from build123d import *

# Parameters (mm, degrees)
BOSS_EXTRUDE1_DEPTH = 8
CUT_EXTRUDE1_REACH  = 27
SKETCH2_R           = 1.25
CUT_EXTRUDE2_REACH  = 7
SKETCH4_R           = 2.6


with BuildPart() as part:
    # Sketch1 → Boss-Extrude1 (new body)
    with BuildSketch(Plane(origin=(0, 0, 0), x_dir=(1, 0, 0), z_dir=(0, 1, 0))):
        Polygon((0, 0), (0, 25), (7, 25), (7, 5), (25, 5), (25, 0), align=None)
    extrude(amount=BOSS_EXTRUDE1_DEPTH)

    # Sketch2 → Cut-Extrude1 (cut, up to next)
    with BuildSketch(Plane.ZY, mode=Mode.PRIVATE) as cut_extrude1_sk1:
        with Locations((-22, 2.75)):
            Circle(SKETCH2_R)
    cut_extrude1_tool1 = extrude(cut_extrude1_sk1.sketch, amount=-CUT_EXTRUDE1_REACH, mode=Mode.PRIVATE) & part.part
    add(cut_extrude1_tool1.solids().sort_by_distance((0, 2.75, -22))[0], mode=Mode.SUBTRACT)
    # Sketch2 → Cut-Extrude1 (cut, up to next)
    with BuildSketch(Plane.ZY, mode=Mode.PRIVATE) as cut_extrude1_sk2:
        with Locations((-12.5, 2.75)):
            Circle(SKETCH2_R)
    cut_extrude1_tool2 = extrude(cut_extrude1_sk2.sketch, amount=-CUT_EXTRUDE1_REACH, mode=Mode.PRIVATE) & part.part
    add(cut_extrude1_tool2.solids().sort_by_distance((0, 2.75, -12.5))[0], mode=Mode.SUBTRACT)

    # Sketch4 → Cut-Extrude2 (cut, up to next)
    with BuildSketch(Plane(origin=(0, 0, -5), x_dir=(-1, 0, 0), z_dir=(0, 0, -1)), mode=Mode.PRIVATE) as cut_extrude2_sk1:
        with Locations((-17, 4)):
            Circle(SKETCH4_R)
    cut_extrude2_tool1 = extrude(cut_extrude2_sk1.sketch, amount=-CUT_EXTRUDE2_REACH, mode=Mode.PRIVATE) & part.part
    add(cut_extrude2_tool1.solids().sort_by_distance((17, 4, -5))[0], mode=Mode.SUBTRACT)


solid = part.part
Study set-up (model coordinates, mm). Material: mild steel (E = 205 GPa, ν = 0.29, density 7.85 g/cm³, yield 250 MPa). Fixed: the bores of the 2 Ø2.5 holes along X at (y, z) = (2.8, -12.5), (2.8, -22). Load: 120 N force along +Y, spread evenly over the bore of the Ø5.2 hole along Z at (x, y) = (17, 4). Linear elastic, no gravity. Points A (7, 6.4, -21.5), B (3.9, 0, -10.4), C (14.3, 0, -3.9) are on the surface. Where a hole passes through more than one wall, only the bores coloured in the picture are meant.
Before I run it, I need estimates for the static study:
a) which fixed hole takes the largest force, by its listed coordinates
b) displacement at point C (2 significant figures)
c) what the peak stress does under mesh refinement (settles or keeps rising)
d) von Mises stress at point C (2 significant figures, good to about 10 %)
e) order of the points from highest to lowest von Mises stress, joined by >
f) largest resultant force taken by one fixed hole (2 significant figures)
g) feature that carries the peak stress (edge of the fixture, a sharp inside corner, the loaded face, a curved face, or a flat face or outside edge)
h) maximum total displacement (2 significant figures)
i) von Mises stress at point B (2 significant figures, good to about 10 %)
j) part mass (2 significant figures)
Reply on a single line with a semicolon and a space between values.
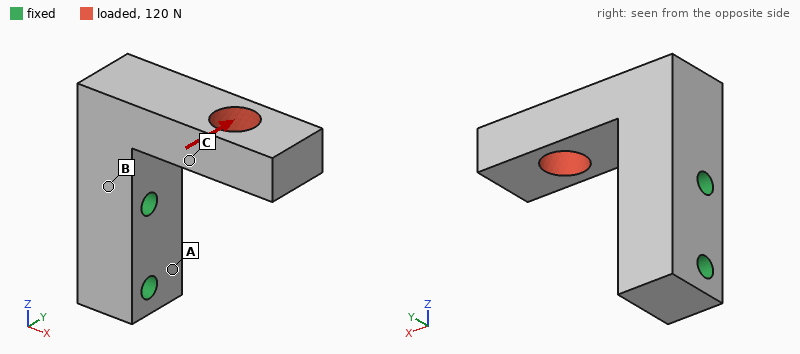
(2.8, -12.5); 7.3 µm; keeps rising; 18 MPa; B > C > A; 190 N; edge of the fixture; 15 µm; 33 MPa; 15 g
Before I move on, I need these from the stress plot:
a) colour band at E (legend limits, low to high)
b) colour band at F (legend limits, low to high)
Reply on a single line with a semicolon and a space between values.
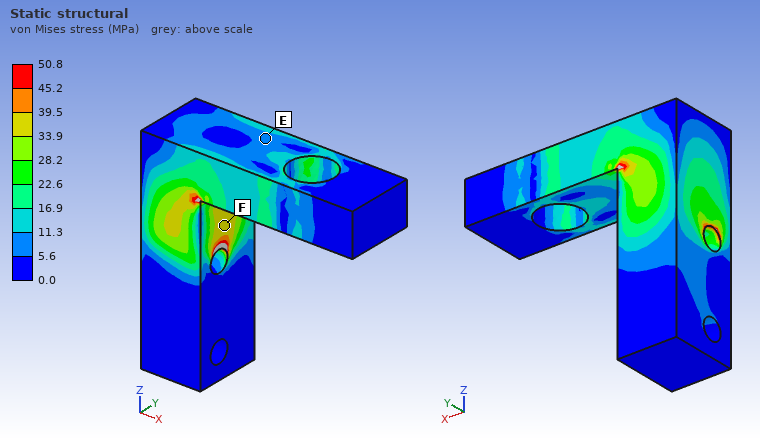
5.6 to 11.3 MPa; 33.9 to 39.5 MPa
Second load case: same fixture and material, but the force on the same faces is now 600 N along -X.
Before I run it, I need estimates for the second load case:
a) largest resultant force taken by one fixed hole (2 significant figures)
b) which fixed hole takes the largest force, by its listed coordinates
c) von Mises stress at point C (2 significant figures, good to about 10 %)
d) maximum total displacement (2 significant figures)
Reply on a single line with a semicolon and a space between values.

690 N; (2.8, -12.5); 23 MPa; 18 µm
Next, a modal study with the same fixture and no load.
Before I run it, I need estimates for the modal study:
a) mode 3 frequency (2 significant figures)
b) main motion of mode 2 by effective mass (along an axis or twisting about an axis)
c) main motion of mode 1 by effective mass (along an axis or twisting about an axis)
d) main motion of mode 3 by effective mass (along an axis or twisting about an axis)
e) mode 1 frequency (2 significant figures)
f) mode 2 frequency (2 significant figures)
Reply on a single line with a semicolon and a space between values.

21 kHz; along Y; along Z; along X; 7400 Hz; 8000 Hz
